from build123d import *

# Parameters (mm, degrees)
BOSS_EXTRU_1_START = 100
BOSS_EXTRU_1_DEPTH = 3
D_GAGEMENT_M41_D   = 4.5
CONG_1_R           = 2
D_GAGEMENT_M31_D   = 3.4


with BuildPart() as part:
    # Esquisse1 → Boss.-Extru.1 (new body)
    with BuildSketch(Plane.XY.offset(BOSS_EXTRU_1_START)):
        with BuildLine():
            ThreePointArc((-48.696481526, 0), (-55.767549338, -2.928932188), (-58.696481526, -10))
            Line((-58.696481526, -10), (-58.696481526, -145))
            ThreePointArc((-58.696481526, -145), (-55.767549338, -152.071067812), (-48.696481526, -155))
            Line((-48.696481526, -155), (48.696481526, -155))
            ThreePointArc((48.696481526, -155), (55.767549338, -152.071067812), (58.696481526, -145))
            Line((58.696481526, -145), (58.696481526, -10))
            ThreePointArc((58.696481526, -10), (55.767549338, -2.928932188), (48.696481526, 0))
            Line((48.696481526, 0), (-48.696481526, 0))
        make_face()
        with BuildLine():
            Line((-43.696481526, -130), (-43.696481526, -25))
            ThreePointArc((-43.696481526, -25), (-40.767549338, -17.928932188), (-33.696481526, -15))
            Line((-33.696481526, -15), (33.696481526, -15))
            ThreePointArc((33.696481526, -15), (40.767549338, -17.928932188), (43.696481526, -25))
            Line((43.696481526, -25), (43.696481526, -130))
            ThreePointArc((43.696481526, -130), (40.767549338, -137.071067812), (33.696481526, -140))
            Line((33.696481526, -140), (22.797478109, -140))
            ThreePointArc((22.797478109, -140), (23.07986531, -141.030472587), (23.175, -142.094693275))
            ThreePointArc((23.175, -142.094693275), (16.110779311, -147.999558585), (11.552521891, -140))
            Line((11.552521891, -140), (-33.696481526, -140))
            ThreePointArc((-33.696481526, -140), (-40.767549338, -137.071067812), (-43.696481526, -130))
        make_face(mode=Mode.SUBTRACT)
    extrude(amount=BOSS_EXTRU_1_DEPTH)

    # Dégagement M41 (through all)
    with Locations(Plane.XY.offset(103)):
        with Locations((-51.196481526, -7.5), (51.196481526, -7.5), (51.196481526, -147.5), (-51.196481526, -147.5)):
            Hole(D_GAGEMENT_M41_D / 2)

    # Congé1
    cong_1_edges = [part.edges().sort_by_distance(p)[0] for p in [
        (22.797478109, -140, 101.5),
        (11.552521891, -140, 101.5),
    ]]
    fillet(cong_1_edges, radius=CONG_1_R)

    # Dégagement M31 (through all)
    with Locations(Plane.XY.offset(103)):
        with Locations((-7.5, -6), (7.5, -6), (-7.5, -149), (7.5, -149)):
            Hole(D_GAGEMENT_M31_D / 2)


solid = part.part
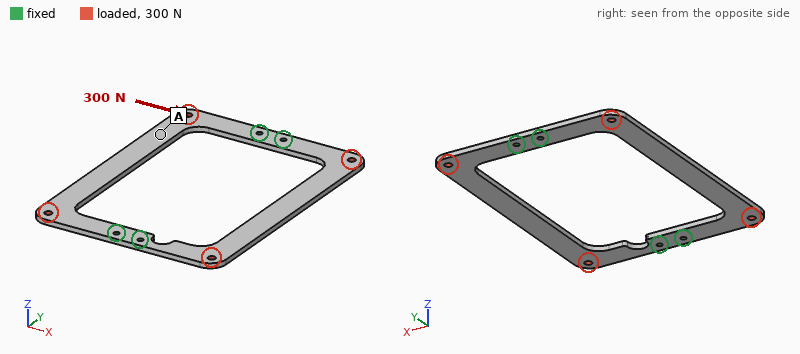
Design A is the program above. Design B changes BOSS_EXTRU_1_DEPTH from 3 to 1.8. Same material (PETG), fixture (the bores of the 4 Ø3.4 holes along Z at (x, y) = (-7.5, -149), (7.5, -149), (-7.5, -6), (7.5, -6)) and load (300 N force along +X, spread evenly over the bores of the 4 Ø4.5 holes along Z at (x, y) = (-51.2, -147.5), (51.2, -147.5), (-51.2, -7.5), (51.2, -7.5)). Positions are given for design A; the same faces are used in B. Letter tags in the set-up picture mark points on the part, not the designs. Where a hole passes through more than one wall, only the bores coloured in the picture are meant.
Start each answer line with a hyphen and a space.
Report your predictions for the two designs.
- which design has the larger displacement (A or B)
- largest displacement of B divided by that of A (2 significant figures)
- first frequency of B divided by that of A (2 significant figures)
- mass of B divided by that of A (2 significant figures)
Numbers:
- B
- 1.7
- 0.61
- 0.60
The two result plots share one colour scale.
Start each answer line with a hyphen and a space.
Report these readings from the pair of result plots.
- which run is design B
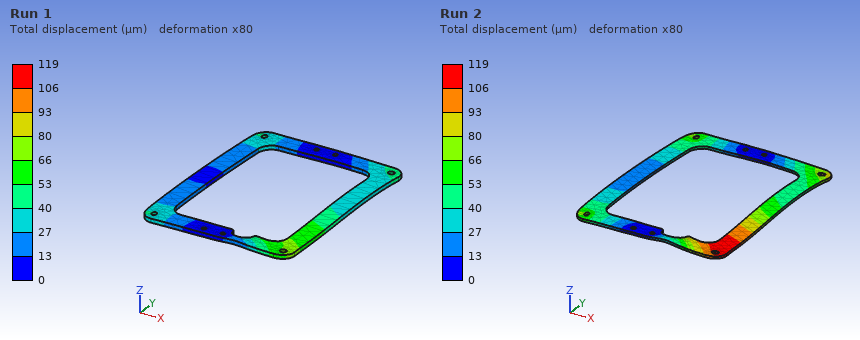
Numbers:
- Run 2
